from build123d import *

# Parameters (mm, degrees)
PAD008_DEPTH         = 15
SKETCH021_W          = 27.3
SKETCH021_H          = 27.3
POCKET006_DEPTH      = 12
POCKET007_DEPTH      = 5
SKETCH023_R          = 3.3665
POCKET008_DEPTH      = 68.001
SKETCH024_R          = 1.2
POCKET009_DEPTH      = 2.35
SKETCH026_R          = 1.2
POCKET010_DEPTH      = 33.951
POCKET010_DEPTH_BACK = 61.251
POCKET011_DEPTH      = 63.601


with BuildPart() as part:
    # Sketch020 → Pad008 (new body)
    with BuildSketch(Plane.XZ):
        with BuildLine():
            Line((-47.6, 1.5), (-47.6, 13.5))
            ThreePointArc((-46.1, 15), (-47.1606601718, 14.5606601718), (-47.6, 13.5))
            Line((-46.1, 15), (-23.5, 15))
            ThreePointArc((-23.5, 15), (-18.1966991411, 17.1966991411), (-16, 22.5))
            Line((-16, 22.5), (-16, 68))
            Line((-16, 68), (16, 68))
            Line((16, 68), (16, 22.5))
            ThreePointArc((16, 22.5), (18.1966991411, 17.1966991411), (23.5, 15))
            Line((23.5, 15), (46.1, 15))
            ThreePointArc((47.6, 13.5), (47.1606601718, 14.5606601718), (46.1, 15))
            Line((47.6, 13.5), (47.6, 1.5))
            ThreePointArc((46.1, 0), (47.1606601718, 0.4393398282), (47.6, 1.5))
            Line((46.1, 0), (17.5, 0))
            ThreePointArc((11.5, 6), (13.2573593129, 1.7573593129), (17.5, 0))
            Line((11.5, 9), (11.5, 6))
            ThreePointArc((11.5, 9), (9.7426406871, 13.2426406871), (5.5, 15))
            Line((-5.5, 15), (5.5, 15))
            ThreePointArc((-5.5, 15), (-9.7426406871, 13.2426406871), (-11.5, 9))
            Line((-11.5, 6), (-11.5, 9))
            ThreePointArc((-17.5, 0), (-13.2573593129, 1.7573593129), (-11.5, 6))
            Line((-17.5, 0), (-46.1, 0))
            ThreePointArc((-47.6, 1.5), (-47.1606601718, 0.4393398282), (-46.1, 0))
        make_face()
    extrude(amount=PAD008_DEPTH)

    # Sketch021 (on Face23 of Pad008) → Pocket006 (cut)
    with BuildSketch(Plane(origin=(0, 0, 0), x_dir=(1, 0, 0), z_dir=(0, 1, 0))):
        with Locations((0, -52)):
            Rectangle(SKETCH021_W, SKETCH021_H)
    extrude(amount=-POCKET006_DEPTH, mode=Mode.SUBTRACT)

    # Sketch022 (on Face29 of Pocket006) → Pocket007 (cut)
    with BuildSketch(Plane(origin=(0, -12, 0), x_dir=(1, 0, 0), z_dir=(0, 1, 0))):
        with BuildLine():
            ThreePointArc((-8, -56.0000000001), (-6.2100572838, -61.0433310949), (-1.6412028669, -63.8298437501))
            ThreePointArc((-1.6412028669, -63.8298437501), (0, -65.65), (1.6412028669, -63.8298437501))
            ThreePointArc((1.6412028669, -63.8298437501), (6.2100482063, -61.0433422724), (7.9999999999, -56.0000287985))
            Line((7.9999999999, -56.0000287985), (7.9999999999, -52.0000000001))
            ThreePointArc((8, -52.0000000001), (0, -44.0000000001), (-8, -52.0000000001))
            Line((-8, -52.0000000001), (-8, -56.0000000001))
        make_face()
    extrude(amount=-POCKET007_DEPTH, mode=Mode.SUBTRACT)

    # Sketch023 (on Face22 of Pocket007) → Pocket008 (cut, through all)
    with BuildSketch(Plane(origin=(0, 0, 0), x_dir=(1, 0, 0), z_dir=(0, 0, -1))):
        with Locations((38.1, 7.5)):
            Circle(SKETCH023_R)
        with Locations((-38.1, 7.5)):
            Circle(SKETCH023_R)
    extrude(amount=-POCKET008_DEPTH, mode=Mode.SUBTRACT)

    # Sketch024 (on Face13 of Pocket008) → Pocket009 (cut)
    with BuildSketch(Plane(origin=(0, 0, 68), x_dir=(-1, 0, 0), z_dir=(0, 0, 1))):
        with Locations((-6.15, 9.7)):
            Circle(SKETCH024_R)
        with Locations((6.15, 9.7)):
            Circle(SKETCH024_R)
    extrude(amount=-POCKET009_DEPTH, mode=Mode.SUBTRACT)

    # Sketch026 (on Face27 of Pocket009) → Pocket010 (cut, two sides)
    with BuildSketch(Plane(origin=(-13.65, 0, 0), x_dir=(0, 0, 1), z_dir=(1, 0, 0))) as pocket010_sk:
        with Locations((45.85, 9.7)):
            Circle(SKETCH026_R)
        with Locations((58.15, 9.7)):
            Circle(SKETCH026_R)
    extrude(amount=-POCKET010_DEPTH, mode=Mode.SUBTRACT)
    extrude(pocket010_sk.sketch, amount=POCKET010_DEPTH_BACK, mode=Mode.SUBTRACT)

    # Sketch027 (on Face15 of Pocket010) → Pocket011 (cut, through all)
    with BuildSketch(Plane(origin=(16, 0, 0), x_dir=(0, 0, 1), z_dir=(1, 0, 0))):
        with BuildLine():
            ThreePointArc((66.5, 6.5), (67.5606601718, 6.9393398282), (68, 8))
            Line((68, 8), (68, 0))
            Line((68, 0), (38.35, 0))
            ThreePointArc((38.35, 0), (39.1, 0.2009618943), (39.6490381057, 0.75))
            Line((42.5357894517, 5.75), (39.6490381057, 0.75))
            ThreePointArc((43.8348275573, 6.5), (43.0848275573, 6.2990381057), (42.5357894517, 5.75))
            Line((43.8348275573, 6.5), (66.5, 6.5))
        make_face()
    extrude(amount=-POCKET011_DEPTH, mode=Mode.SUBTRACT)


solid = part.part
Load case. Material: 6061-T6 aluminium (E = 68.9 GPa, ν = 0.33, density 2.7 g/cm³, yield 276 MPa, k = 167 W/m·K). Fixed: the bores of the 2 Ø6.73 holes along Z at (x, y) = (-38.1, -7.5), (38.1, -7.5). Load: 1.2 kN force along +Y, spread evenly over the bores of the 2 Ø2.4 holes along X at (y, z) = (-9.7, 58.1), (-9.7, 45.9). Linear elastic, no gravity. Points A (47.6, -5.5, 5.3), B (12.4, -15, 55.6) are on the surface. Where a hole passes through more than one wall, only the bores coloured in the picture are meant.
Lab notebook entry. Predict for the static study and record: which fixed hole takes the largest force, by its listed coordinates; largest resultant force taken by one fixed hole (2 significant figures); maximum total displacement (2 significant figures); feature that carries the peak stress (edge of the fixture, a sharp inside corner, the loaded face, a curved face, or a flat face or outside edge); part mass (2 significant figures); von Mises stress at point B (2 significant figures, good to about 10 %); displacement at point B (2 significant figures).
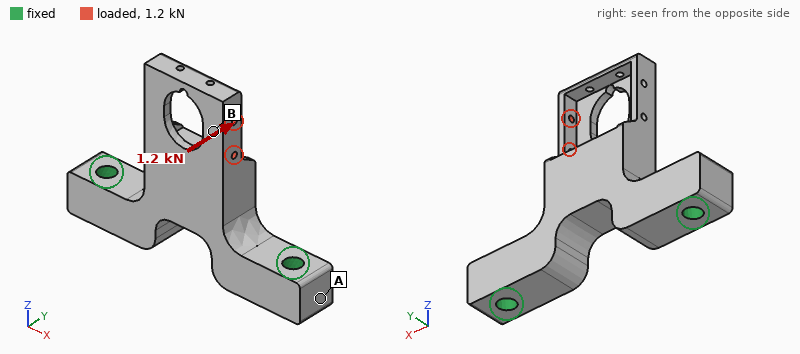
(38.1, -7.5)
910 N
0.60 mm
a curved face
81 g
50 MPa
0.39 mm
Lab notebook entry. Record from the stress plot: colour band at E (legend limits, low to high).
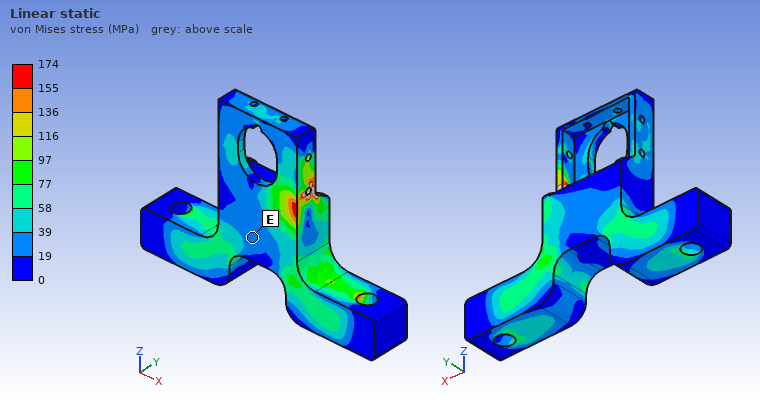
19 to 39 MPa
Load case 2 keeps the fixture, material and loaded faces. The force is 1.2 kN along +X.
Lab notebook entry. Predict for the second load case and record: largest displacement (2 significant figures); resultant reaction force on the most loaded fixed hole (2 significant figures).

0.16 mm
1.3 kN
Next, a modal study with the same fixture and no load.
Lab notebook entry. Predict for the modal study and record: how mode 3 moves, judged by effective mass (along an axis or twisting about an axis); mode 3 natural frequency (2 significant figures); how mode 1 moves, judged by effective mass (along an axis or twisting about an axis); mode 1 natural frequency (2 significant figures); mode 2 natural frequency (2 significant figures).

along Y
6600 Hz
along Y
2700 Hz
5400 Hz
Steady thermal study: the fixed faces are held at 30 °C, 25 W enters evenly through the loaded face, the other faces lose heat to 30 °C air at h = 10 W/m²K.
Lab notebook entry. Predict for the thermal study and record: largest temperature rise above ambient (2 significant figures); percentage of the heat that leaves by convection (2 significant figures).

66 K
6.0 %
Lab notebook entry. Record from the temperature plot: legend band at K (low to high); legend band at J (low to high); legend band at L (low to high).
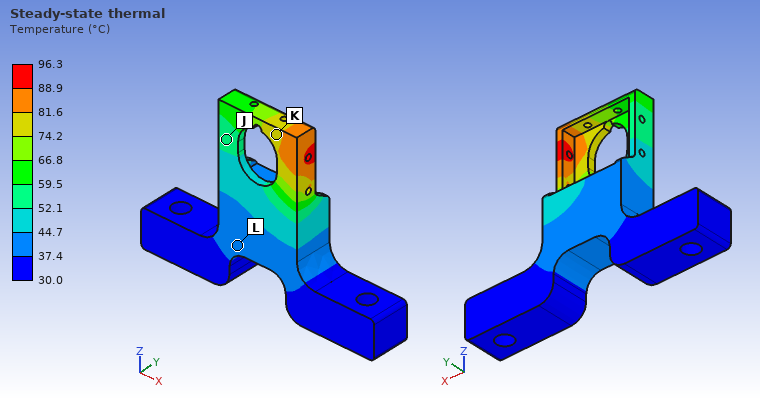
74.2 to 81.6 °C
52.1 to 59.5 °C
37.4 to 44.7 °C
